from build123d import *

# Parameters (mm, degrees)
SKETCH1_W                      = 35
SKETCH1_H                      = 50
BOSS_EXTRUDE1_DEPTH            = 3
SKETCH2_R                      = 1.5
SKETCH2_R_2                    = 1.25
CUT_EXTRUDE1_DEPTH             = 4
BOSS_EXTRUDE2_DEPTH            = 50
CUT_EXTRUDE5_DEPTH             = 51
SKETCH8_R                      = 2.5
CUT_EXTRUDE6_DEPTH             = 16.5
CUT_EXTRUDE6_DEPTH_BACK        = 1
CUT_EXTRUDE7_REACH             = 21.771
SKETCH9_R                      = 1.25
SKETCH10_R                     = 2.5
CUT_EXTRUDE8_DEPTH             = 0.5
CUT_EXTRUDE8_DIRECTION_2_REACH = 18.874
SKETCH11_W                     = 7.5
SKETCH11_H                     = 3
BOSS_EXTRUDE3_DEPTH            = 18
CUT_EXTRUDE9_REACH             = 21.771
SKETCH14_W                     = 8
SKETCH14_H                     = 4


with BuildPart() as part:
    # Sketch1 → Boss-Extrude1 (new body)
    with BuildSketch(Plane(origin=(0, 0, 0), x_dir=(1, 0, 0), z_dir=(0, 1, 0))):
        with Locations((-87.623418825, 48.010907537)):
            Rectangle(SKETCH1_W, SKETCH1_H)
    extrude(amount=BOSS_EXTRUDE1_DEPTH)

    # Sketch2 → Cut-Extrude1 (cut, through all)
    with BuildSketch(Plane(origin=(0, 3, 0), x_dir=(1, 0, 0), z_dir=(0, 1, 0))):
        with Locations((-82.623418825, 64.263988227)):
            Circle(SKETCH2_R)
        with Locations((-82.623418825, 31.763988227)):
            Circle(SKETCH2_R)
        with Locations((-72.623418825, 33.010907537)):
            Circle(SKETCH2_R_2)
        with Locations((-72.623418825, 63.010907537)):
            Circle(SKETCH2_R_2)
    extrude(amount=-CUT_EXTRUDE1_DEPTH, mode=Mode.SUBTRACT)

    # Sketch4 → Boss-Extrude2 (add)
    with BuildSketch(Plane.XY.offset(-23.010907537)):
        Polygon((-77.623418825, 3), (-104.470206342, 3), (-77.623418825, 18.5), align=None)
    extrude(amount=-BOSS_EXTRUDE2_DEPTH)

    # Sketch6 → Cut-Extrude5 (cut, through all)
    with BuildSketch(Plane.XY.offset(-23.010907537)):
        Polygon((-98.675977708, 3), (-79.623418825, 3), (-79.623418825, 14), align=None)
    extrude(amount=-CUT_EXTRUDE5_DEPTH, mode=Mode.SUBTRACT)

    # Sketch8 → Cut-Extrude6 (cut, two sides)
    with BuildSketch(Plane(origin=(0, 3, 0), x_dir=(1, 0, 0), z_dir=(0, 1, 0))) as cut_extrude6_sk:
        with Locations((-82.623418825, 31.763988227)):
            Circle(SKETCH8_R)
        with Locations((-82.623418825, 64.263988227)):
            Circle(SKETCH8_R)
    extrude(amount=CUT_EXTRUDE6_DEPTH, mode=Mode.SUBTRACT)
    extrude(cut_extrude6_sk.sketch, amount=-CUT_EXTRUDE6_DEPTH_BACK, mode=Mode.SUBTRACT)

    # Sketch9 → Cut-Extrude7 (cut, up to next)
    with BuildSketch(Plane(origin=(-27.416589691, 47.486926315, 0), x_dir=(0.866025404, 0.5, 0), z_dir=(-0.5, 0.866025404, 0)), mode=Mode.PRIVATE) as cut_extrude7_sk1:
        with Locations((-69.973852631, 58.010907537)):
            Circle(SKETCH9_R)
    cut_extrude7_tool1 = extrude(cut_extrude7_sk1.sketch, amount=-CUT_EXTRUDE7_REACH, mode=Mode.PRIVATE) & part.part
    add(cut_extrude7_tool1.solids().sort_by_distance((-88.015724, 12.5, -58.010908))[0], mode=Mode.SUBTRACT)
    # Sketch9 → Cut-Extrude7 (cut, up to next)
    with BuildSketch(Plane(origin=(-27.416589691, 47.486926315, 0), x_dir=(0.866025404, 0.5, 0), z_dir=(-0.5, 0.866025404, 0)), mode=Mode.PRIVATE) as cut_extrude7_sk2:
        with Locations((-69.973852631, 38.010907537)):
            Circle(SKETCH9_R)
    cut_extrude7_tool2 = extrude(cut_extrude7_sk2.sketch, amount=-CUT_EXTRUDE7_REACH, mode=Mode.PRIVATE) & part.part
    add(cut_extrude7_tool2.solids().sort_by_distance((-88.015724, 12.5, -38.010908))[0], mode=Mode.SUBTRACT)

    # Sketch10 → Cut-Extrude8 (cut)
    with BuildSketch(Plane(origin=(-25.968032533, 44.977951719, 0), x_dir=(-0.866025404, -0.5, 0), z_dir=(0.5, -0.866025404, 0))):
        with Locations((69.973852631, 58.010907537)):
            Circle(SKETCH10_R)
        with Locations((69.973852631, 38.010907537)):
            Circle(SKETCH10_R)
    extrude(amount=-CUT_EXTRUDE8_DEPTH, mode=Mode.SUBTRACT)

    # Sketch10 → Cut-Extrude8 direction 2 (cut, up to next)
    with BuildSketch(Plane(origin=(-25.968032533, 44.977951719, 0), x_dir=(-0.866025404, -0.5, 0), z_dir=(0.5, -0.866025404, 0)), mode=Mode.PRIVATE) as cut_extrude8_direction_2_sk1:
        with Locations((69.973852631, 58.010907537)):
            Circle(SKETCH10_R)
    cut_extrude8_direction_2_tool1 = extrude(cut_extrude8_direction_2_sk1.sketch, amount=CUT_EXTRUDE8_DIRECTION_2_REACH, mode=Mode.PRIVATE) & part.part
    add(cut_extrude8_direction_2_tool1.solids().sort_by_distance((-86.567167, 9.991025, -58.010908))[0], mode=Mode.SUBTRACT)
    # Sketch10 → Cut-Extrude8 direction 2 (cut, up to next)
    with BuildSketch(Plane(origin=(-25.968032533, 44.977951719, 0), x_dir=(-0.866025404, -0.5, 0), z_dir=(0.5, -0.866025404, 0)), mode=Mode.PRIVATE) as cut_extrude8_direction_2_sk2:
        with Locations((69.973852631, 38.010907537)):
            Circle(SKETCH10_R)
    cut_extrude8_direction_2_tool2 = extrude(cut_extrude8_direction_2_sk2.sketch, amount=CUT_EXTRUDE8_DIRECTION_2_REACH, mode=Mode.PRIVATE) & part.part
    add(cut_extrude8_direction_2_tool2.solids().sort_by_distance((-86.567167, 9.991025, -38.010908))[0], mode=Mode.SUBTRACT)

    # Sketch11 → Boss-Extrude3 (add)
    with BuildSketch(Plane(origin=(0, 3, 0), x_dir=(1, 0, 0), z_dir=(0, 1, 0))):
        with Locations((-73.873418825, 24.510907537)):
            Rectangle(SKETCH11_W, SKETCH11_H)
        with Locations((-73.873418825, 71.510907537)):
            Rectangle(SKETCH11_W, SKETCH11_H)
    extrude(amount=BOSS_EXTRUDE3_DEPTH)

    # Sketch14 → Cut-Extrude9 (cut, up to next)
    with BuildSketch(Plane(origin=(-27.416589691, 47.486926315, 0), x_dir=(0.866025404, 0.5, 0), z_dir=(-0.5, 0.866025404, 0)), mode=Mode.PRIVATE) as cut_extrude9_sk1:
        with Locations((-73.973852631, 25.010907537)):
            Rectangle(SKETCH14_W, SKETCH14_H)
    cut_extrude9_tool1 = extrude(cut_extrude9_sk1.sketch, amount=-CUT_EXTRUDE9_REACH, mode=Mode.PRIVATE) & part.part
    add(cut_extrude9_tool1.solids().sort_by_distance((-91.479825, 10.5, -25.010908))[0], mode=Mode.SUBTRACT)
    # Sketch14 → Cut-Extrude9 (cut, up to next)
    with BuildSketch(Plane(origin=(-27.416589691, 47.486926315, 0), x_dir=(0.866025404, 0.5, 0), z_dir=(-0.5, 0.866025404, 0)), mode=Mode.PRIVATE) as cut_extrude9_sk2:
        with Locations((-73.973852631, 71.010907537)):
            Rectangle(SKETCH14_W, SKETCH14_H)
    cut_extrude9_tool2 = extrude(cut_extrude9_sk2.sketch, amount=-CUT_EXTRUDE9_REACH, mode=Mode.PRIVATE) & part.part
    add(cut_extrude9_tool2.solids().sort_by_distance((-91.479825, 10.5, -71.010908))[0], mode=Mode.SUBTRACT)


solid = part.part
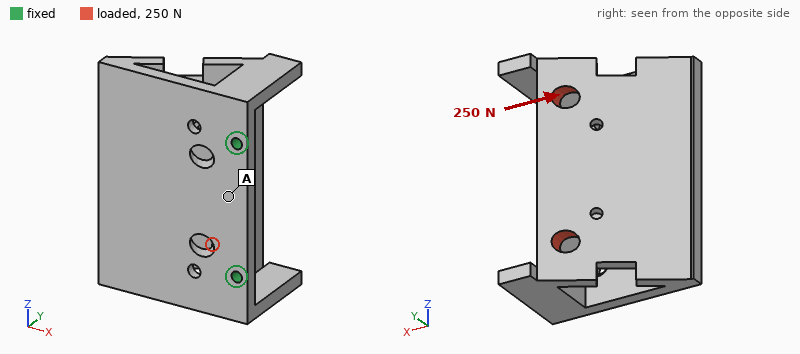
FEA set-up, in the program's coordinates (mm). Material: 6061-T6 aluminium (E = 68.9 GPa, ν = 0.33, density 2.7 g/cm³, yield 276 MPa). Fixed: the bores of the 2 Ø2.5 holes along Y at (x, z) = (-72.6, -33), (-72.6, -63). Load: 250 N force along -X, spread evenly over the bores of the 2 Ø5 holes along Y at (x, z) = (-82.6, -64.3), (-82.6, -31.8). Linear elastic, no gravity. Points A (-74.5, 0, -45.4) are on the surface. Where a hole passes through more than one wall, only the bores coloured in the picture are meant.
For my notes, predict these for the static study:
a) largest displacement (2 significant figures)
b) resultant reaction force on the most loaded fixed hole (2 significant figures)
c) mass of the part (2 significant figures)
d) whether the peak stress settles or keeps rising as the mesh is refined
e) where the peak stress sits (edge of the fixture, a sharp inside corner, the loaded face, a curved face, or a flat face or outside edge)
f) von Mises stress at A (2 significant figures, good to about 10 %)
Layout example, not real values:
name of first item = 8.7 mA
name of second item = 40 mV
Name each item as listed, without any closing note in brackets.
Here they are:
largest displacement = 0.11 mm
resultant reaction force on the most loaded fixed hole = 130 N
mass of the part = 29 g
whether the peak stress settles or keeps rising as the mesh is refined = keeps rising
where the peak stress sits = edge of the fixture
von Mises stress at A = 10.0 MPa
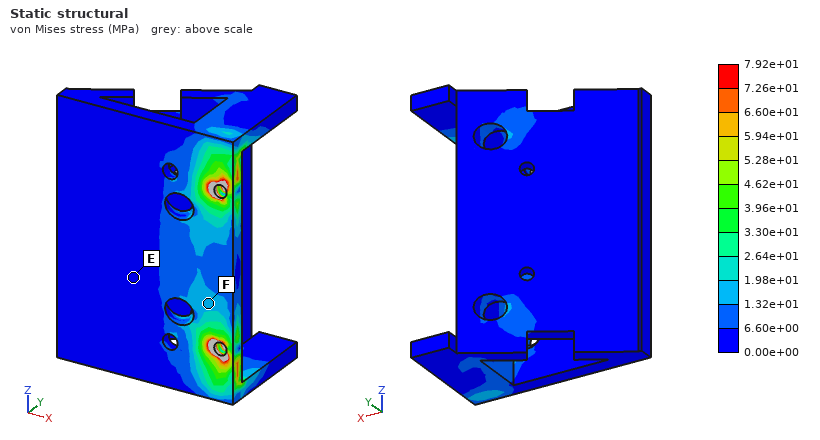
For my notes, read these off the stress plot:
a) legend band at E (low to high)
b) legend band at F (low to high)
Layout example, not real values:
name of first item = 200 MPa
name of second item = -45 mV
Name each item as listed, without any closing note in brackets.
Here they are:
legend band at E = 0.00e+00 to 6.60e+00 MPa
legend band at F = 1.32e+01 to 1.98e+01 MPa
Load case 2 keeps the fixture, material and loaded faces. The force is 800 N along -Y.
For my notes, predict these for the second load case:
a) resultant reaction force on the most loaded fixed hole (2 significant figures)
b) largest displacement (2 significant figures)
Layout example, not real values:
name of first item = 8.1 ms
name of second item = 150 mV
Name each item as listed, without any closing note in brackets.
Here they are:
resultant reaction force on the most loaded fixed hole = 400 N
largest displacement = 0.23 mm
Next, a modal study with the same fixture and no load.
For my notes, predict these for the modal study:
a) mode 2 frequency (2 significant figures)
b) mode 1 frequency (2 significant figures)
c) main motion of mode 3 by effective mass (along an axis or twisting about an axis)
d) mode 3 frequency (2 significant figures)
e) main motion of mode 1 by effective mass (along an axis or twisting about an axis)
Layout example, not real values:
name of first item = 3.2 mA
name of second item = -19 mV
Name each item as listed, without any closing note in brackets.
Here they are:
mode 2 frequency = 6500 Hz
mode 1 frequency = 1600 Hz
main motion of mode 3 by effective mass = along Z
mode 3 frequency = 8700 Hz
main motion of mode 1 by effective mass = along Y
